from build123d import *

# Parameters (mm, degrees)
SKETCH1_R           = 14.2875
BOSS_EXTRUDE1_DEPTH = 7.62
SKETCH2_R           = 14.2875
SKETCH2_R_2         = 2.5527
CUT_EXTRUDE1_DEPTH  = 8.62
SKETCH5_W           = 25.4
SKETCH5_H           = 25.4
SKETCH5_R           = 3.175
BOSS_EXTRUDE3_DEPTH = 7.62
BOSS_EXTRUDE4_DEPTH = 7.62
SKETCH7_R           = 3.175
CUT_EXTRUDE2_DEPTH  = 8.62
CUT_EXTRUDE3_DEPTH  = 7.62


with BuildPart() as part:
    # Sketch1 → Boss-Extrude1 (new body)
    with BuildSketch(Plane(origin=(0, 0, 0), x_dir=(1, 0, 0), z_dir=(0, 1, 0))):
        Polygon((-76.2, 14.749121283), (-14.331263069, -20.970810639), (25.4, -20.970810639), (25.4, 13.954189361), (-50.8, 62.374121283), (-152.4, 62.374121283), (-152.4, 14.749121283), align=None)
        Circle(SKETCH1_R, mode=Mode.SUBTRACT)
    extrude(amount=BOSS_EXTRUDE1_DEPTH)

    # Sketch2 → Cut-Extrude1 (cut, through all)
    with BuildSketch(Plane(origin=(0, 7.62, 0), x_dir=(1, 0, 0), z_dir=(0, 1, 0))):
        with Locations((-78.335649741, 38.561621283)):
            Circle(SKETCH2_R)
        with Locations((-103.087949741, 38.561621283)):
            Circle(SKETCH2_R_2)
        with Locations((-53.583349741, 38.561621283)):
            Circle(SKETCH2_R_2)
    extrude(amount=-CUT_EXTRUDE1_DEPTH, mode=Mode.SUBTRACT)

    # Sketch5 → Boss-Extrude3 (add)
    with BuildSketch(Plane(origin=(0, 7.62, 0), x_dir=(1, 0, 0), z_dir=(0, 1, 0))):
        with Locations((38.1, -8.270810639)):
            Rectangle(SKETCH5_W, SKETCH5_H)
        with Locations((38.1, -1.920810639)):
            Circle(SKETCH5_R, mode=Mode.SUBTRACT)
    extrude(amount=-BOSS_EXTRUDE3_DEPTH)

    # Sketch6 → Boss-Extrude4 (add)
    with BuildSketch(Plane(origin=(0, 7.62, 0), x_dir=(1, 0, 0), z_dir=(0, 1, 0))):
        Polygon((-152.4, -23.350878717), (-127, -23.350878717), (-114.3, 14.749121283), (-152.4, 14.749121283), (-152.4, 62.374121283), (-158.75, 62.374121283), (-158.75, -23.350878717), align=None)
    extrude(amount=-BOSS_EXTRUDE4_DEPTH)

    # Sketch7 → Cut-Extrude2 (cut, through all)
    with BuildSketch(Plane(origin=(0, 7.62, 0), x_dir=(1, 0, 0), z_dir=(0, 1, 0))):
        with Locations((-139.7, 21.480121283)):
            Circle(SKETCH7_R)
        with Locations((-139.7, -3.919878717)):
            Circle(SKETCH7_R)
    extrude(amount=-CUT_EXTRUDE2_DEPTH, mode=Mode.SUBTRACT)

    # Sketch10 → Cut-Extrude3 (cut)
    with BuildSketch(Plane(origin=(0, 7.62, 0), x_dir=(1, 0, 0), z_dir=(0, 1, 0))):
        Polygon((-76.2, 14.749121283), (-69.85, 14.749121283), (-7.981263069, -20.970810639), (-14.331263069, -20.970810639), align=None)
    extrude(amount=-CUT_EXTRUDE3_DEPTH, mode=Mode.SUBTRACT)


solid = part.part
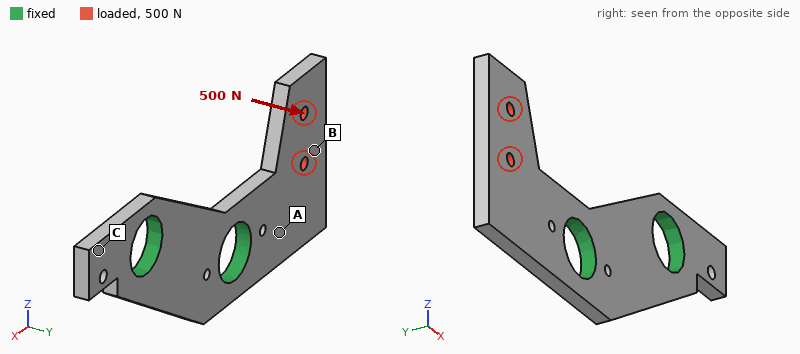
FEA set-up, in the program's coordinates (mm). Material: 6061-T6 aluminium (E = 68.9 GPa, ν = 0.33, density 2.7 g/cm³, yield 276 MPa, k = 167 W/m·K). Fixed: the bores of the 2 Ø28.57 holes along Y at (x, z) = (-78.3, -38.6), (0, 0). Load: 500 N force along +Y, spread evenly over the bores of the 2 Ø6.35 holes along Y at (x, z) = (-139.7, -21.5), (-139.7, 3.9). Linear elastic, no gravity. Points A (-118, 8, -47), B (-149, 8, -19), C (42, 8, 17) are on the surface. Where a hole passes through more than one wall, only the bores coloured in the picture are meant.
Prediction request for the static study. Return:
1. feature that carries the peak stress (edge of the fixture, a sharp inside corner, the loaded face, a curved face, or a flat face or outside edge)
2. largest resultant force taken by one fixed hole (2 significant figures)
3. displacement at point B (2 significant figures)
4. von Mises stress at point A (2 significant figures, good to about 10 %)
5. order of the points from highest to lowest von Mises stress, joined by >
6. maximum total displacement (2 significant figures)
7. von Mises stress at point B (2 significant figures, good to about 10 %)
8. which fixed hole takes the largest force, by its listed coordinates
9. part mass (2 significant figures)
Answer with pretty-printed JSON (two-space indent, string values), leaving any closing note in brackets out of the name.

{
  "feature that carries the peak stress": "a curved face",
  "largest resultant force taken by one fixed hole": "500 N",
  "displacement at point B": "0.28 mm",
  "von Mises stress at point A": "31 MPa",
  "order of the points from highest to lowest von Mises stress, joined by >": "A > B > C",
  "maximum total displacement": "0.50 mm",
  "von Mises stress at point B": "11 MPa",
  "which fixed hole takes the largest force, by its listed coordinates": "(-78.3, -38.6)",
  "part mass": "200 g"
}
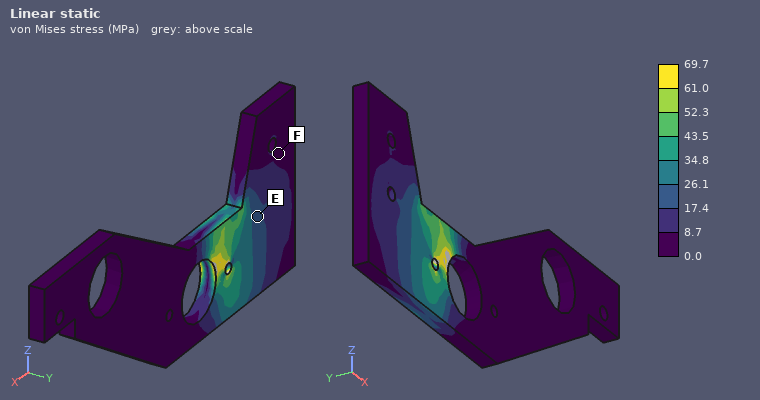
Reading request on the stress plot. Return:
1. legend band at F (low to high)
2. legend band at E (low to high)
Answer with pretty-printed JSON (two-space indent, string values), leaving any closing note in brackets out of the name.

{
  "legend band at F": "0.0 to 8.7 MPa",
  "legend band at E": "17.4 to 26.1 MPa"
}
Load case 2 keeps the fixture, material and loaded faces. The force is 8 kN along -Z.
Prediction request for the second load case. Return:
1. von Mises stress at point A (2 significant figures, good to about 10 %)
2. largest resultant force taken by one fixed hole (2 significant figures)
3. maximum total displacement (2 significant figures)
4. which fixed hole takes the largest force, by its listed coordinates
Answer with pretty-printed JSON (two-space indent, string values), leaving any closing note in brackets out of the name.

{
  "von Mises stress at point A": "53 MPa",
  "largest resultant force taken by one fixed hole": "8.4 kN",
  "maximum total displacement": "0.32 mm",
  "which fixed hole takes the largest force, by its listed coordinates": "(-78.3, -38.6)"
}
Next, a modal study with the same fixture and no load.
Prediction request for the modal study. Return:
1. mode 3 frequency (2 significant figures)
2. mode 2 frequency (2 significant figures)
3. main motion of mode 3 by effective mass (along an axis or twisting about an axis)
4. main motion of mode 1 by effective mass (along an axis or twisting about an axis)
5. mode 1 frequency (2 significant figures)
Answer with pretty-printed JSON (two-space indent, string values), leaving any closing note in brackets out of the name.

{
  "mode 3 frequency": "3500 Hz",
  "mode 2 frequency": "1800 Hz",
  "main motion of mode 3 by effective mass": "along Z",
  "main motion of mode 1 by effective mass": "along Y",
  "mode 1 frequency": "890 Hz"
}
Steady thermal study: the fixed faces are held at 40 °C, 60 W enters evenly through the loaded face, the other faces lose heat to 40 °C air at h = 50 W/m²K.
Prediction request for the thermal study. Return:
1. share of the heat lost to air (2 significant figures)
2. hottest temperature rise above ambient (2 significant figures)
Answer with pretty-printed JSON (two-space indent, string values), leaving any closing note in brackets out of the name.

{
  "share of the heat lost to air": "29 %",
  "hottest temperature rise above ambient": "53 K"
}
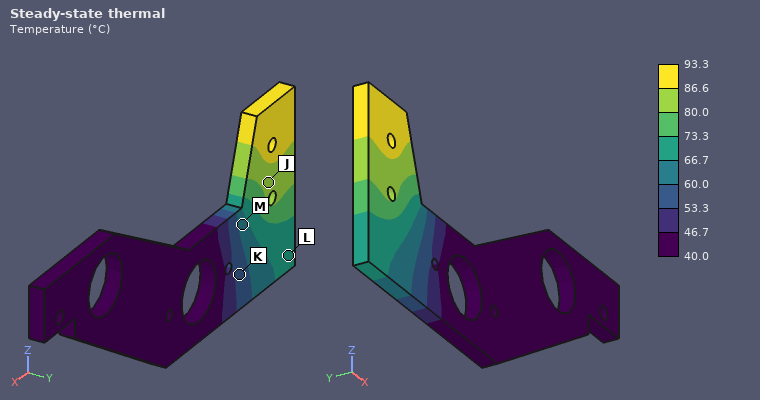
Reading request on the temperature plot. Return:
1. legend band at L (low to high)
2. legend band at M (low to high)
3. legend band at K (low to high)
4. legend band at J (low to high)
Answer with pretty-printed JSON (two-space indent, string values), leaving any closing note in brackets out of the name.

{
  "legend band at L": "66.7 to 73.3 °C",
  "legend band at M": "60.0 to 66.7 °C",
  "legend band at K": "53.3 to 60.0 °C",
  "legend band at J": "80.0 to 86.6 °C"
}
